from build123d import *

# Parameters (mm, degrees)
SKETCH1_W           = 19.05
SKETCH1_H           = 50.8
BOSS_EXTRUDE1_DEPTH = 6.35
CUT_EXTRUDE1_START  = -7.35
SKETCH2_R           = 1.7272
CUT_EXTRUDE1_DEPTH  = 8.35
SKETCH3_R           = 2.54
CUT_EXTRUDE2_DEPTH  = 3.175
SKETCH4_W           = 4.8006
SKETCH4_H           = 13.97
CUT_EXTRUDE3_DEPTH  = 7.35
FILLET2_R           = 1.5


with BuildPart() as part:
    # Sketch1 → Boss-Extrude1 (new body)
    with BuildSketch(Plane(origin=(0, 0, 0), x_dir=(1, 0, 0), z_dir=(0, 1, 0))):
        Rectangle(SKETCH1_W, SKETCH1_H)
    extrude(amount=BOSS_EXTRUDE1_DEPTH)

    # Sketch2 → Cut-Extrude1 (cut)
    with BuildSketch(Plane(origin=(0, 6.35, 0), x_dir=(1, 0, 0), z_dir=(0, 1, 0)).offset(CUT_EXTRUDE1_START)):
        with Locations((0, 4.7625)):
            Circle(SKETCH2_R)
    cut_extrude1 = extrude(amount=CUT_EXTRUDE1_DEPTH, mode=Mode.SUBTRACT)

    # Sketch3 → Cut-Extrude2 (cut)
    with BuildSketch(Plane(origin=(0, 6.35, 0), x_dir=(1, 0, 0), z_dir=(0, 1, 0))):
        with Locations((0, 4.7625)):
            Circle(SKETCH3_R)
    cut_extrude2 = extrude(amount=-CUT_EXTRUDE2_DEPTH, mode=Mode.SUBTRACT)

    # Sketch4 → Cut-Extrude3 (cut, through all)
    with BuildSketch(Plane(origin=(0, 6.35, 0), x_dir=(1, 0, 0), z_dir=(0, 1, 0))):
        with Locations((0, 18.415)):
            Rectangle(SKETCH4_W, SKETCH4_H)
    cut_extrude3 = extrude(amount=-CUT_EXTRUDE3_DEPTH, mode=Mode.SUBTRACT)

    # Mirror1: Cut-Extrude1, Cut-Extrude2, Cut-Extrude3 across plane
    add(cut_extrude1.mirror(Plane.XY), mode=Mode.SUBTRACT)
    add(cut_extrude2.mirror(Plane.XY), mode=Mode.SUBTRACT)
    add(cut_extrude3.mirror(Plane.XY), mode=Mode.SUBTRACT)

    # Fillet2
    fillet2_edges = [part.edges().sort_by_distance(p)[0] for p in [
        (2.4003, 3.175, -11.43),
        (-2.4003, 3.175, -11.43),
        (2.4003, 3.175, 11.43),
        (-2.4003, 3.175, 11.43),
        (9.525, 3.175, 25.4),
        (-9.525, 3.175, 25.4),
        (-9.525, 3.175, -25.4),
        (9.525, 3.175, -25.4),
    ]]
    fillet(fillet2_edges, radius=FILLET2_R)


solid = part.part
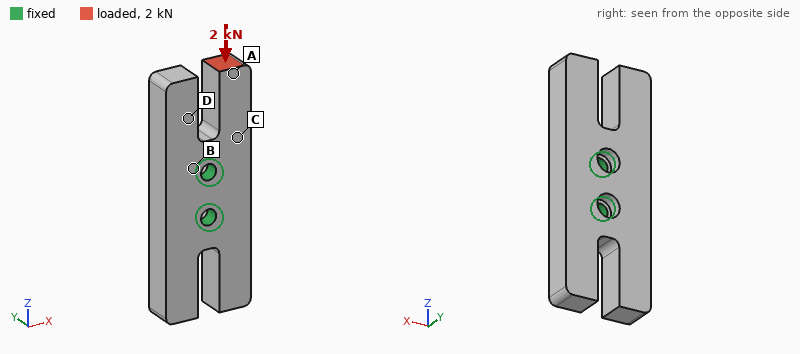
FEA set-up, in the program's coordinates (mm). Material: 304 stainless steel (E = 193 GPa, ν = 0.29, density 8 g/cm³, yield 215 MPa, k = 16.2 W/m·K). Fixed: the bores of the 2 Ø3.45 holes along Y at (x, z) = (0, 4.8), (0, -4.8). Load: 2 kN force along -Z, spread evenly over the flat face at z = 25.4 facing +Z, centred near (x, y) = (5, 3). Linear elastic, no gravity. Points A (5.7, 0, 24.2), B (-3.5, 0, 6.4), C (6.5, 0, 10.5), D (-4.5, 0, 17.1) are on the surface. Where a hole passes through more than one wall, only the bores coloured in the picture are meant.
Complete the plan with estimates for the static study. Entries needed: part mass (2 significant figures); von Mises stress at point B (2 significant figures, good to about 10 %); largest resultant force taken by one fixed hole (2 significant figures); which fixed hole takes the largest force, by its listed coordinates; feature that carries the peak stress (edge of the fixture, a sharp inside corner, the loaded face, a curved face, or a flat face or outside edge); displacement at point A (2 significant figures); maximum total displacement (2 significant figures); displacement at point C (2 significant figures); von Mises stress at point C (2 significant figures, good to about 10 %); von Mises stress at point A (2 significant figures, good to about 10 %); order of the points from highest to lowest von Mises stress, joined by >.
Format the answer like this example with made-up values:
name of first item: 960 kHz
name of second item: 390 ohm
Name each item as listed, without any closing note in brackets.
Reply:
part mass: 41 g
von Mises stress at point B: 18 MPa
largest resultant force taken by one fixed hole: 1.5 kN
which fixed hole takes the largest force, by its listed coordinates: (0, 4.8)
feature that carries the peak stress: edge of the fixture
displacement at point A: 7.0 µm
maximum total displacement: 8.8 µm
displacement at point C: 3.6 µm
von Mises stress at point C: 36 MPa
von Mises stress at point A: 55 MPa
order of the points from highest to lowest von Mises stress, joined by >: A > C > B > D
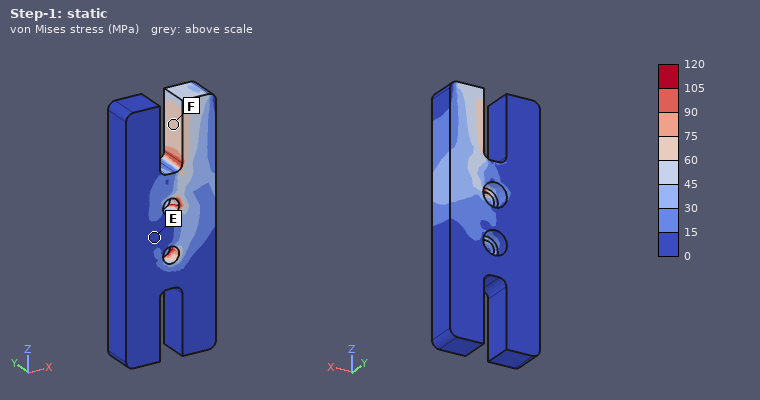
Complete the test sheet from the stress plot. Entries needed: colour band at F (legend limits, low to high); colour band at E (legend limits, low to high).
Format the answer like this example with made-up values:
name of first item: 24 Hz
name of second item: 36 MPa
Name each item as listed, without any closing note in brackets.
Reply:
colour band at F: 60 to 75 MPa
colour band at E: 0 to 15 MPa
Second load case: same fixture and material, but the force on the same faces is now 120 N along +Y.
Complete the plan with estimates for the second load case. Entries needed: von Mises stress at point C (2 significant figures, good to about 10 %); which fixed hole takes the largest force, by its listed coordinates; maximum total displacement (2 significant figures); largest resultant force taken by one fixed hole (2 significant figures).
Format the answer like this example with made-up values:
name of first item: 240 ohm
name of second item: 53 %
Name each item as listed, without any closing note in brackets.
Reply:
von Mises stress at point C: 31 MPa
which fixed hole takes the largest force, by its listed coordinates: (0, 4.8)
maximum total displacement: 15 µm
largest resultant force taken by one fixed hole: 310 N
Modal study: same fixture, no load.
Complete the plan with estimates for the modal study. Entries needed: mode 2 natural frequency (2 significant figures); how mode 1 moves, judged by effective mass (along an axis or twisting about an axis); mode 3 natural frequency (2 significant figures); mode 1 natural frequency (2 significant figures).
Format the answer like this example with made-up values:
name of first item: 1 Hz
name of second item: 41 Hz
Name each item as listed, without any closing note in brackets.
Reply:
mode 2 natural frequency: 9900 Hz
how mode 1 moves, judged by effective mass: twisting about X
mode 3 natural frequency: 10 kHz
mode 1 natural frequency: 9000 Hz
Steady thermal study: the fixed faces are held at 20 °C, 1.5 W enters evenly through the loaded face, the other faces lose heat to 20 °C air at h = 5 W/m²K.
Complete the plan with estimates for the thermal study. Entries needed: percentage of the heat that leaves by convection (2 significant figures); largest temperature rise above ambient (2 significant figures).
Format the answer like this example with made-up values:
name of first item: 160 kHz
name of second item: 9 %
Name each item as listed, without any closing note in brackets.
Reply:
percentage of the heat that leaves by convection: 5.1 %
largest temperature rise above ambient: 42 K
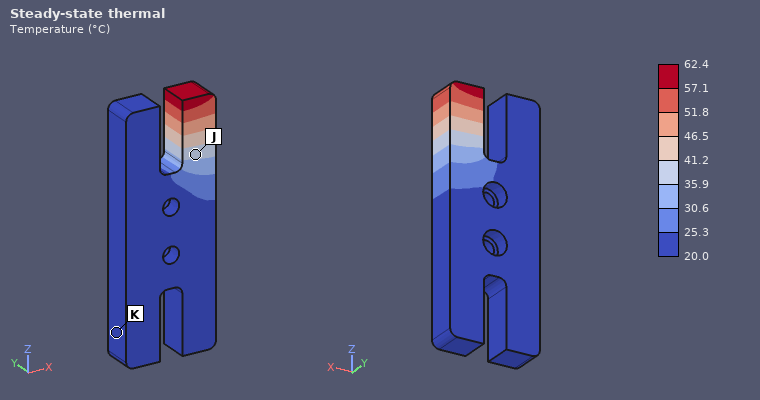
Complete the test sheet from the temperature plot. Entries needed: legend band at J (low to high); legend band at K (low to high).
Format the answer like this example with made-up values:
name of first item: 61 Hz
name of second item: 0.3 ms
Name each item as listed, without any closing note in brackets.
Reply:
legend band at J: 35.9 to 41.2 °C
legend band at K: 20.0 to 25.3 °C
